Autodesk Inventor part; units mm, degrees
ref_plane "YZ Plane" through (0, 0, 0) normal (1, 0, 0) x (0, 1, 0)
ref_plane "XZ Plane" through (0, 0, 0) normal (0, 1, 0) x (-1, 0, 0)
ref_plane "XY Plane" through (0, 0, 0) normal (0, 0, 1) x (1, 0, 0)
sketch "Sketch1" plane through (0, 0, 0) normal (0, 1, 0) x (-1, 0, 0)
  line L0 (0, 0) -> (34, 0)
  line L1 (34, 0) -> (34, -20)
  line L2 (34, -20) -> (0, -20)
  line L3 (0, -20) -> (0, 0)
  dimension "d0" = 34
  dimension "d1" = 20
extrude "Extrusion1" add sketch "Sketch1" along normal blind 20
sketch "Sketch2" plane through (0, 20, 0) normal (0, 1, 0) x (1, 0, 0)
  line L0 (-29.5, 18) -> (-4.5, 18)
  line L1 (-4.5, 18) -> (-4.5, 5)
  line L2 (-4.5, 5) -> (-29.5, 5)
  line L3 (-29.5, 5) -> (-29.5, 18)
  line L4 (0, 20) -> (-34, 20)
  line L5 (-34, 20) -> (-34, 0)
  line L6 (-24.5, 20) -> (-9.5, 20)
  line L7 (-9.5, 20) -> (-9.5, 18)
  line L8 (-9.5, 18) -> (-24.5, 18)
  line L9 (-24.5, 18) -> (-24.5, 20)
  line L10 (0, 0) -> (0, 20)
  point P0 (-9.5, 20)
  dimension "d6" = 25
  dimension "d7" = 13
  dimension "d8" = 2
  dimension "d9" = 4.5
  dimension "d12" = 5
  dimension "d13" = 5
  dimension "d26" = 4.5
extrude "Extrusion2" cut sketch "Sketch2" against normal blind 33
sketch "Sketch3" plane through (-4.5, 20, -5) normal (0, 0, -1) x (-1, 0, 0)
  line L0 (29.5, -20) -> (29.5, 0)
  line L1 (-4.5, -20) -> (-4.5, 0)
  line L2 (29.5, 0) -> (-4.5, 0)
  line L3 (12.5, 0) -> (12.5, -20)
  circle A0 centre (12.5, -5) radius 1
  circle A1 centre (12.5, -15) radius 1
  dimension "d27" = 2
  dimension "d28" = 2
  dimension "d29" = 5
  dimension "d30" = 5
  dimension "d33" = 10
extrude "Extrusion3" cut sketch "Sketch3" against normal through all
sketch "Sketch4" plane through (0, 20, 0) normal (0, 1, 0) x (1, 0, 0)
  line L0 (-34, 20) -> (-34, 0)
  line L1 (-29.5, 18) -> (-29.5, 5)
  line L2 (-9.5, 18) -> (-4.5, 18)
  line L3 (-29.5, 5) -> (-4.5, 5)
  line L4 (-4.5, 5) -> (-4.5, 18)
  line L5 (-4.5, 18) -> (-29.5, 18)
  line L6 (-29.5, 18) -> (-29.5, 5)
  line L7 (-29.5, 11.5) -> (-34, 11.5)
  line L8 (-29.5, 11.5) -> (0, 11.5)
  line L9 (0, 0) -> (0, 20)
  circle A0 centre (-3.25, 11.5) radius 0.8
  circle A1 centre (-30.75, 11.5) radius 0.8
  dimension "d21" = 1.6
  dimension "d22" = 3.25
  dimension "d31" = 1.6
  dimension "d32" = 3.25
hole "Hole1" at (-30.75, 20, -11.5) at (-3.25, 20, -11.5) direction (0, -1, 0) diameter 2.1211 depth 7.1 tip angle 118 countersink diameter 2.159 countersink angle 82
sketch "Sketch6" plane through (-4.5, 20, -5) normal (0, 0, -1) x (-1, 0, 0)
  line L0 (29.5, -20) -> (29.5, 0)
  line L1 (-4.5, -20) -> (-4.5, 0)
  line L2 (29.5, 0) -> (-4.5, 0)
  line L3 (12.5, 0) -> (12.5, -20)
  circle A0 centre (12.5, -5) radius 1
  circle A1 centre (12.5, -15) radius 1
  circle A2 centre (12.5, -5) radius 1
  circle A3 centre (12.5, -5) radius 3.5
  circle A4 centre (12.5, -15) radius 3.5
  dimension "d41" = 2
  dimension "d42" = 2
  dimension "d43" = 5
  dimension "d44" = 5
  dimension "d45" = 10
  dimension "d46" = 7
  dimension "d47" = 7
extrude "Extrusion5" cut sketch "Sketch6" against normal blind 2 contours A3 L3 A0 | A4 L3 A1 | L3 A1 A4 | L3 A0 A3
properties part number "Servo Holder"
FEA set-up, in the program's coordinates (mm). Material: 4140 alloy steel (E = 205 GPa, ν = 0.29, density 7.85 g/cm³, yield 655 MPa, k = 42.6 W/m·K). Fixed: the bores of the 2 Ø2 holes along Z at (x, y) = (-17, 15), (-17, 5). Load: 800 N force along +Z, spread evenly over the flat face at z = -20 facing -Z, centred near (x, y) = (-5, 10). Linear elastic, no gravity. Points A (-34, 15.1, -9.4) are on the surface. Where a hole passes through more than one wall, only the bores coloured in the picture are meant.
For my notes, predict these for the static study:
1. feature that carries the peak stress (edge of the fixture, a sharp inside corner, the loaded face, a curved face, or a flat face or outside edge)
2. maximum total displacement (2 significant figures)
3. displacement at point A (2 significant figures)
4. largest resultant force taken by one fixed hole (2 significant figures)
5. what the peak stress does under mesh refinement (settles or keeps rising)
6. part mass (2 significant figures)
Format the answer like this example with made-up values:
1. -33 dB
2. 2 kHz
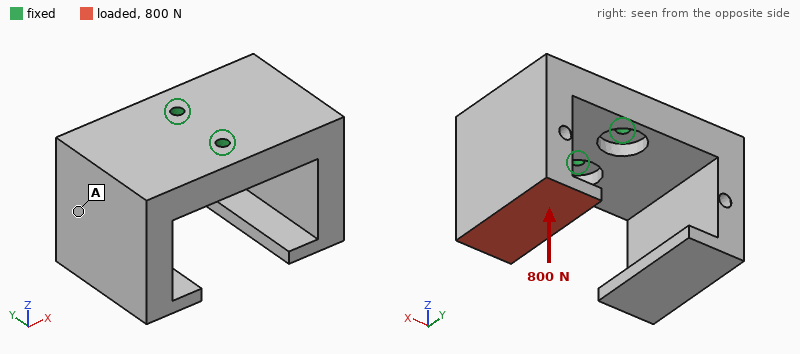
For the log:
1. edge of the fixture
2. 68 µm
3. 24 µm
4. 400 N
5. keeps rising
6. 49 g
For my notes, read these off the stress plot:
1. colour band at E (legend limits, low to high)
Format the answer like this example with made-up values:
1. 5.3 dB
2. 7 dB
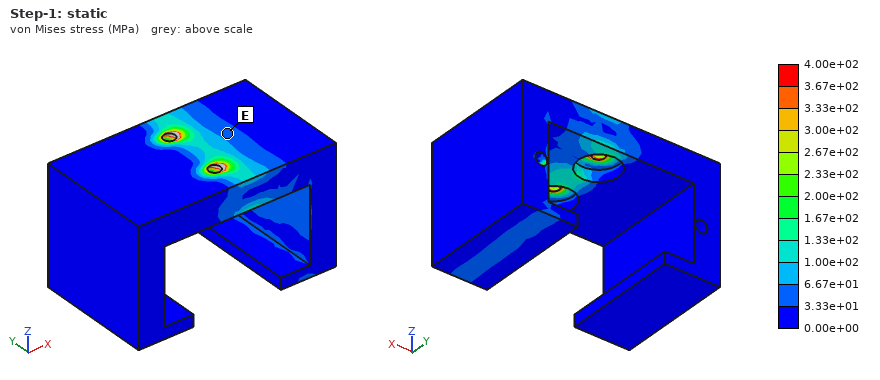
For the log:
1. 3.33e+01 to 6.67e+01 MPa
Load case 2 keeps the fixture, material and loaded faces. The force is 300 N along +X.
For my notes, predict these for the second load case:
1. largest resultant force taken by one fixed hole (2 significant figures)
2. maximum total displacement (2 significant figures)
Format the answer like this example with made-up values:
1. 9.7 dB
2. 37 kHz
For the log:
1. 150 N
2. 76 µm
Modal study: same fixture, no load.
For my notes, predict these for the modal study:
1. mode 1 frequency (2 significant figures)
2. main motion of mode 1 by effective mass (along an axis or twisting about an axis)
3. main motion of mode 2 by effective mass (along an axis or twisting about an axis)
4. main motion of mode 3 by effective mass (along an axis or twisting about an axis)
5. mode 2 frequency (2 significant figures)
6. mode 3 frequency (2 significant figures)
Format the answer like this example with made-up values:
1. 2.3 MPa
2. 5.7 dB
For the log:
1. 3000 Hz
2. along X
3. along Z
4. twisting about Z
5. 4400 Hz
6. 6600 Hz
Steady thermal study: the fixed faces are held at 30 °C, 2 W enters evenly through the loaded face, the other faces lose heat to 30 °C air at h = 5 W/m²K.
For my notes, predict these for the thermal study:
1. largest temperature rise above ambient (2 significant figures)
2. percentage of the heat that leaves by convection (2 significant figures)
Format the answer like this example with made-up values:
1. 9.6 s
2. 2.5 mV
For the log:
1. 18 K
2. 4.4 %
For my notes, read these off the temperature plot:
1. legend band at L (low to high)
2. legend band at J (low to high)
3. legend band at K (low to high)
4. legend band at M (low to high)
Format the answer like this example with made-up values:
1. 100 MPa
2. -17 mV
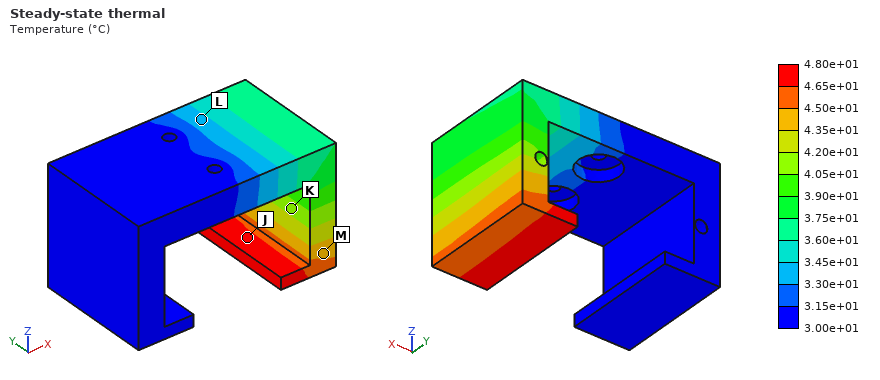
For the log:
1. 3.30e+01 to 3.45e+01 °C
2. 4.65e+01 to 4.80e+01 °C
3. 4.05e+01 to 4.20e+01 °C
4. 4.35e+01 to 4.50e+01 °C
